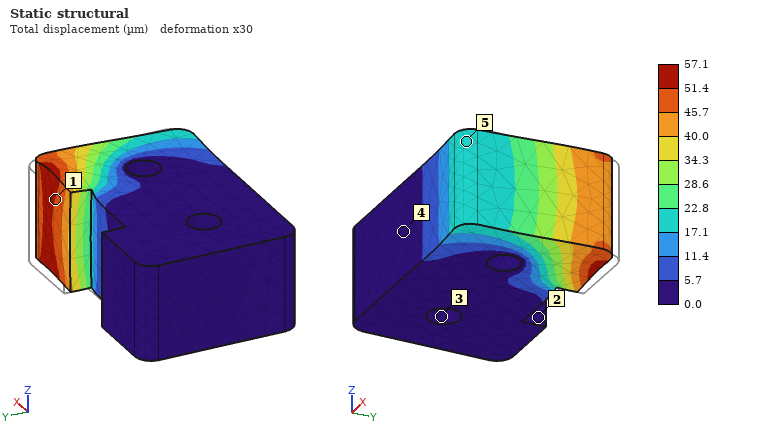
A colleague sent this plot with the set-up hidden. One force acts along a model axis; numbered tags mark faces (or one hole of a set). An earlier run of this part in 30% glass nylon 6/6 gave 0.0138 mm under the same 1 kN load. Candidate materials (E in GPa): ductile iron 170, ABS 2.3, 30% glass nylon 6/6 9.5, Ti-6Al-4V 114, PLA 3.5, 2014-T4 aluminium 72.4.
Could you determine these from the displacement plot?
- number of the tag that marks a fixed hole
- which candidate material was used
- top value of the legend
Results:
3
ABS
57.1 µm
